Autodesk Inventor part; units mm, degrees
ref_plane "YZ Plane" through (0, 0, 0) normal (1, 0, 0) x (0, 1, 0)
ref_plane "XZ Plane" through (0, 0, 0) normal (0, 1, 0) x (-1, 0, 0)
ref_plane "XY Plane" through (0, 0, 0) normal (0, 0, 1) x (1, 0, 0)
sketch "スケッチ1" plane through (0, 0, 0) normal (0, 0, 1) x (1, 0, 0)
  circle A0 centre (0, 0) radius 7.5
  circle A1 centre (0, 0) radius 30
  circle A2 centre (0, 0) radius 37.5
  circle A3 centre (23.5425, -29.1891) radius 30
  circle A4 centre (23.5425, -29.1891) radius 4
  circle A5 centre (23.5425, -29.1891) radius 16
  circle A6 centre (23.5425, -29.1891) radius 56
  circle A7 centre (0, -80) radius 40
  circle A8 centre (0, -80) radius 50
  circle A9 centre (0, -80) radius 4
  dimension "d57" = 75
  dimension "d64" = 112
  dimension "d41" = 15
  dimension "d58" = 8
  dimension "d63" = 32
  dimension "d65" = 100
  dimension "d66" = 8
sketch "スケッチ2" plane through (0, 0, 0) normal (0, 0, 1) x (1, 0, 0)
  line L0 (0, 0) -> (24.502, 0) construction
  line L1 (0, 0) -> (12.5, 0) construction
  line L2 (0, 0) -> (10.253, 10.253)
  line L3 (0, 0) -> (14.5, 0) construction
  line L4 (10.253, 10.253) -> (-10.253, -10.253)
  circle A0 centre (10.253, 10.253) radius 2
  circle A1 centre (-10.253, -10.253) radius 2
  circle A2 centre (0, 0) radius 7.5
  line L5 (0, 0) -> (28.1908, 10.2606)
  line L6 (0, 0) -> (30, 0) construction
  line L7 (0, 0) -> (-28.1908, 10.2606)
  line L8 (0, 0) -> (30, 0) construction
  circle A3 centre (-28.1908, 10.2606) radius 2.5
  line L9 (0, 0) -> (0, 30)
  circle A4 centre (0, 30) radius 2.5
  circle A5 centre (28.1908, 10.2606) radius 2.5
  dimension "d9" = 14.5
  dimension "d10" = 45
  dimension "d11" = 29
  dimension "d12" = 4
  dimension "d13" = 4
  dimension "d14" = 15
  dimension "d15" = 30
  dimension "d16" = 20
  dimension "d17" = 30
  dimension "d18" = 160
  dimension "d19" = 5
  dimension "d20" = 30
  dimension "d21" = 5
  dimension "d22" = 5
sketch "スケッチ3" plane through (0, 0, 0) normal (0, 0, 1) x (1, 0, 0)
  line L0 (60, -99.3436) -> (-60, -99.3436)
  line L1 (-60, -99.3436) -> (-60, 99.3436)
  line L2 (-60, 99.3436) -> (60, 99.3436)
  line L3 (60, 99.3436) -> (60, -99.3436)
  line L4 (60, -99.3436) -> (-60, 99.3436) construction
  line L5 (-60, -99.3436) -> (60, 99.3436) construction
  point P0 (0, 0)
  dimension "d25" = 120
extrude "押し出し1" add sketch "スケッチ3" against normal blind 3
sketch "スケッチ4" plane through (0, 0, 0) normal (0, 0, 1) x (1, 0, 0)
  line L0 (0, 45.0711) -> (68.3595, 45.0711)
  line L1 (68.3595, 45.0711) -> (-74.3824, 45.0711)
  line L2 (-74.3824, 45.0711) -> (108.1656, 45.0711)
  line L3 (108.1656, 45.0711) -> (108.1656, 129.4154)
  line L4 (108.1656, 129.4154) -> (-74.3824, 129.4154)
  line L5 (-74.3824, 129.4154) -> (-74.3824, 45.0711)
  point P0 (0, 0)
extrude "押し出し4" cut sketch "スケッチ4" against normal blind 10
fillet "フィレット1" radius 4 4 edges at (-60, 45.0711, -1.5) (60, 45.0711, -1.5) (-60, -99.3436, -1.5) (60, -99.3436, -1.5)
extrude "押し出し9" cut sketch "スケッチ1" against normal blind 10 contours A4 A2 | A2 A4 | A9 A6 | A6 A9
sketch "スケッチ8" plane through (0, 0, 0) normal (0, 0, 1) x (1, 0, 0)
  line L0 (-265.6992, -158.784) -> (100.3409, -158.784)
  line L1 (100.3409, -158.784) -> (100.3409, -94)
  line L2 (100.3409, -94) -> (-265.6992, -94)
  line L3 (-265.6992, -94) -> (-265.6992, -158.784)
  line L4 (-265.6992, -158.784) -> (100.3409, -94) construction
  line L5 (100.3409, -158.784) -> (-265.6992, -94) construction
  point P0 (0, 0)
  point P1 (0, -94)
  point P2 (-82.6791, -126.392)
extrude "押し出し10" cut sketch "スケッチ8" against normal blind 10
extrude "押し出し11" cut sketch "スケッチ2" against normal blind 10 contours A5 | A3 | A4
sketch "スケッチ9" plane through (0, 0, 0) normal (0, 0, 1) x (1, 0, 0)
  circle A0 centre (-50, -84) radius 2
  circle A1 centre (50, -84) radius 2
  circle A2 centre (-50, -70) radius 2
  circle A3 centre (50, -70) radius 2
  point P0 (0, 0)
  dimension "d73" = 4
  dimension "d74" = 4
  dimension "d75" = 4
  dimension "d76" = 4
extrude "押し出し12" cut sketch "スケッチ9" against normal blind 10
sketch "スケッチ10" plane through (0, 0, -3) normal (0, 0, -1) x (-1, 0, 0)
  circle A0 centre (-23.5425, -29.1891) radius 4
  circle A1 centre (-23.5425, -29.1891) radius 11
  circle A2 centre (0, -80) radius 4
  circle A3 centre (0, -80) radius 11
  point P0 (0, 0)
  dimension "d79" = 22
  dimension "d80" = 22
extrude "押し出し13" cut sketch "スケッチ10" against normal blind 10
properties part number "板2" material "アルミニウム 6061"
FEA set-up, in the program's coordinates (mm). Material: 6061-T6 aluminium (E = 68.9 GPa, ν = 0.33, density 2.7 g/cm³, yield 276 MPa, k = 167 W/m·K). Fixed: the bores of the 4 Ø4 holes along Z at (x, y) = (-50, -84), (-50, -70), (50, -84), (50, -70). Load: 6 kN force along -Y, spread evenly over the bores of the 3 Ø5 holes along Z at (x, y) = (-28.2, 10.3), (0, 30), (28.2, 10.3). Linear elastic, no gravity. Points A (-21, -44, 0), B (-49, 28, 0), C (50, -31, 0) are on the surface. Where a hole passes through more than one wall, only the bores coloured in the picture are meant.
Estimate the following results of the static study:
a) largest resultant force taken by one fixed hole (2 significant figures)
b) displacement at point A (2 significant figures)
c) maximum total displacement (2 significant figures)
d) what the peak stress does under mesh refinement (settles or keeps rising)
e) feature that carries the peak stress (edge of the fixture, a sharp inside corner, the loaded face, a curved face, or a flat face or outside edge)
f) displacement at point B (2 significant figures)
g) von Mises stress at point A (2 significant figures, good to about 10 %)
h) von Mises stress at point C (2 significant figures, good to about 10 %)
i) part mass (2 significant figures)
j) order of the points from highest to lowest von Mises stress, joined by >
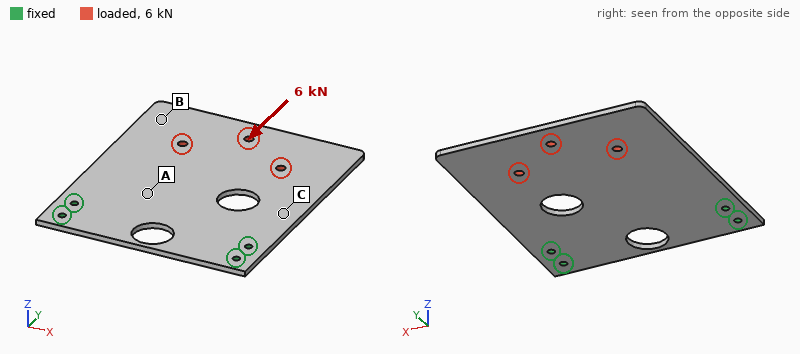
2.1 kN
21 µm
46 µm
keeps rising
edge of the fixture
27 µm
16 MPa
25 MPa
130 g
C > A > B
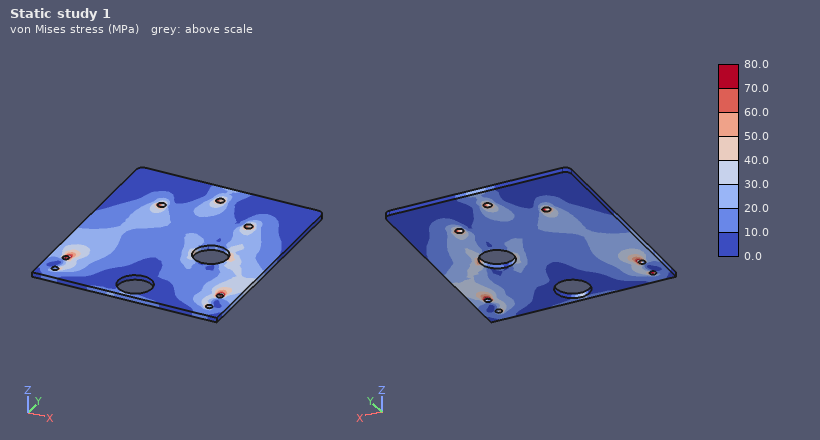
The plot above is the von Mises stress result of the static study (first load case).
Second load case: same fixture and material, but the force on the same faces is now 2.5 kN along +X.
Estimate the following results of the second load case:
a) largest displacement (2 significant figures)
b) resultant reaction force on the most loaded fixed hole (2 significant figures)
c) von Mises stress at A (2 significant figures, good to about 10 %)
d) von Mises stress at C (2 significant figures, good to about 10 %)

73 µm
1.9 kN
17 MPa
20 MPa
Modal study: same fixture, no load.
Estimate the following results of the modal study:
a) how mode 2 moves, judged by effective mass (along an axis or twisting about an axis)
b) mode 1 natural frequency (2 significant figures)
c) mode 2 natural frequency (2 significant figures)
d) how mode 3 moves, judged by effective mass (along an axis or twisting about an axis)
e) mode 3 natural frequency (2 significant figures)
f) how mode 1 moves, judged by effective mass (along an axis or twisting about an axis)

twisting about Y
160 Hz
430 Hz
along Z
1000 Hz
along Z
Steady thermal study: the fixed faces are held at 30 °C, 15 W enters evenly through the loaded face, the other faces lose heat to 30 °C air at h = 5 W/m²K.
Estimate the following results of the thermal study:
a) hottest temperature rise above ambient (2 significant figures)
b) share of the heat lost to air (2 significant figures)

28 K
16 %
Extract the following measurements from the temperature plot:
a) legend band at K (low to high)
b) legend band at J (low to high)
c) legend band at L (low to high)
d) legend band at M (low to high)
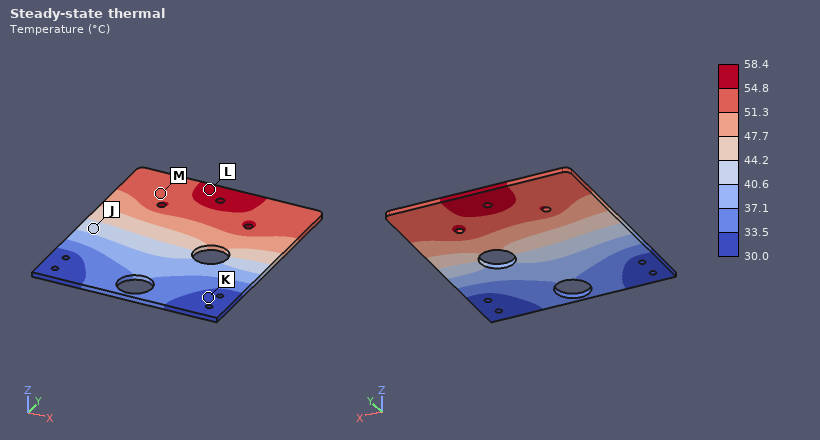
30.0 to 33.5 °C
40.6 to 44.2 °C
54.8 to 58.4 °C
51.3 to 54.8 °C
